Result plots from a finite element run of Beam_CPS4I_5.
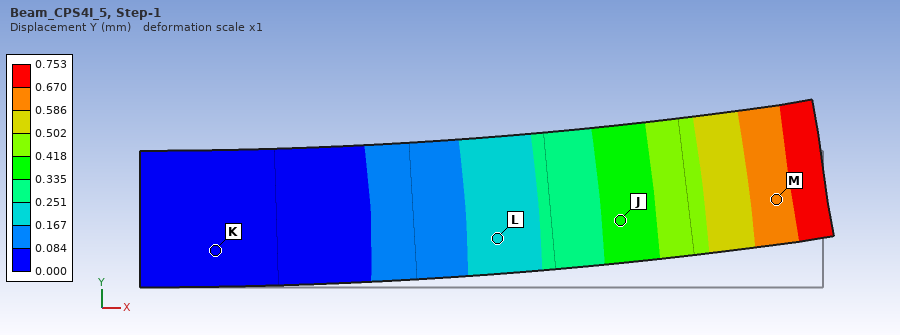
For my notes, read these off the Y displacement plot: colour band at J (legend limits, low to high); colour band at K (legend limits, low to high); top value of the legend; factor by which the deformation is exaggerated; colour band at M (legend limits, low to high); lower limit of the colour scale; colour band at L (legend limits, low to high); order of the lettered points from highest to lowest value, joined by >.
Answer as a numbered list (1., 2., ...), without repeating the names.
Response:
1. 0.335 to 0.418 mm
2. 0.000 to 0.084 mm
3. 0.753 mm
4. 1
5. 0.586 to 0.670 mm
6. 0.000 mm
7. 0.167 to 0.251 mm
8. M > J > L > K
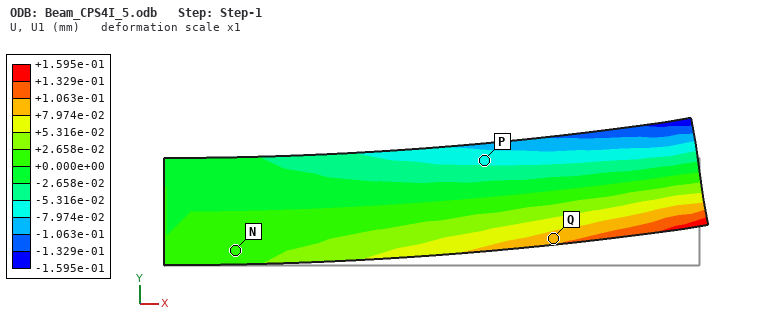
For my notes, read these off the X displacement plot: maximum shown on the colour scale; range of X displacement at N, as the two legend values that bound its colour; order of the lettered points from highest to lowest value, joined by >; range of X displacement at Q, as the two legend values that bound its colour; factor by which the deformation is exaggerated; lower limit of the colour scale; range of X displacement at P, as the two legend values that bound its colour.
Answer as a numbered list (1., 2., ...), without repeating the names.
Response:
1. +1.595e-01 mm
2. +0.000e+00 to +2.658e-02 mm
3. Q > N > P
4. +7.974e-02 to +1.063e-01 mm
5. 1
6. -1.595e-01 mm
7. -7.974e-02 to -5.316e-02 mm
